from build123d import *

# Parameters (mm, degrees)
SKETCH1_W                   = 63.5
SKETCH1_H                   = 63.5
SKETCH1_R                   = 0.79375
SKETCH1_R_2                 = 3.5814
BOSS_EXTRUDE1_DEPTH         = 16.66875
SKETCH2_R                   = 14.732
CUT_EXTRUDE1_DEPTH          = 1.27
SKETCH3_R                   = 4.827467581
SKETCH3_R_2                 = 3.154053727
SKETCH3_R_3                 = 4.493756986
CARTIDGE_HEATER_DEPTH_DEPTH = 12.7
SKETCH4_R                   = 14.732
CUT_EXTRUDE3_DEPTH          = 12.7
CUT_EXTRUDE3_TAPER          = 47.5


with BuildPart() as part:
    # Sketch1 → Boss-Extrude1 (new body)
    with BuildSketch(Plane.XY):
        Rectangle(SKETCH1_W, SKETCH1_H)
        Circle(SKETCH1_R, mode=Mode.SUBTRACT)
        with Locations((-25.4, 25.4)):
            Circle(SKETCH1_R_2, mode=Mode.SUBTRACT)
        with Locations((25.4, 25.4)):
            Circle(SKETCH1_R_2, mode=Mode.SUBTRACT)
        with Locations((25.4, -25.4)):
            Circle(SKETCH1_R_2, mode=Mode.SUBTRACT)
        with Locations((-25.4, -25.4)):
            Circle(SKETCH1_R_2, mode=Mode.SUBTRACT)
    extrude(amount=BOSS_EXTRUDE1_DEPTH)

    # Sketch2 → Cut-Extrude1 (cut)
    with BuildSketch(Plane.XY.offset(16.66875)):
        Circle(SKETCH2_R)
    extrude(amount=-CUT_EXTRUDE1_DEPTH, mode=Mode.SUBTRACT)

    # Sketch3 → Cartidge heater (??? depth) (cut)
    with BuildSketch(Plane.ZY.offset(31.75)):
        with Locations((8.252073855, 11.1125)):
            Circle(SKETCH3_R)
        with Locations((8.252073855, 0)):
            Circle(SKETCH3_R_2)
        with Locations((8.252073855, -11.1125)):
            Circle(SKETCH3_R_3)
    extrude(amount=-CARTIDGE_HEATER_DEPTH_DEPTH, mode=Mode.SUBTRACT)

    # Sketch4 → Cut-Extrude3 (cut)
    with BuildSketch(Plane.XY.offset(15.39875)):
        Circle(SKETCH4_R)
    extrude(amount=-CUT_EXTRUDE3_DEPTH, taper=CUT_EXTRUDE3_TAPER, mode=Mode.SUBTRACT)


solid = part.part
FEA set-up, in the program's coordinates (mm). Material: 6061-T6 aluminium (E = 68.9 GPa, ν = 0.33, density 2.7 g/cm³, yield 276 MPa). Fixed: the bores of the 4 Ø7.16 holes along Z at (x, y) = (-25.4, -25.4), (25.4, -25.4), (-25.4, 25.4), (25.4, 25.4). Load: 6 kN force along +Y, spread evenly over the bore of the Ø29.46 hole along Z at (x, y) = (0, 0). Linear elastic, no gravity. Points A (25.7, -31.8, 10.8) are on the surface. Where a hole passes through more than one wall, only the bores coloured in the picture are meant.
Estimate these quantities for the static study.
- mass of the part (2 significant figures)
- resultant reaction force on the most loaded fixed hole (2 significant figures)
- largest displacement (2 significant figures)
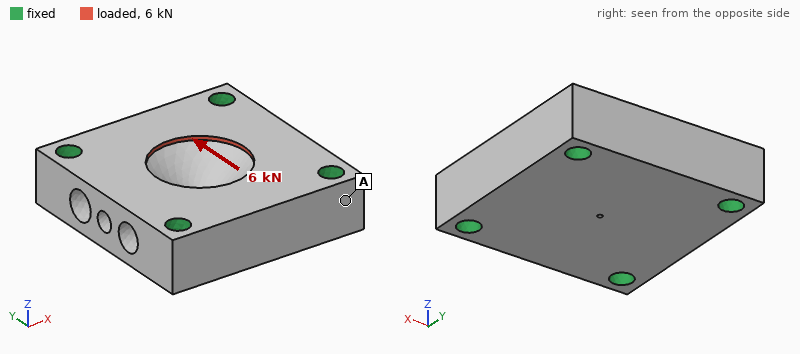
160 g
1.8 kN
5.9 µm
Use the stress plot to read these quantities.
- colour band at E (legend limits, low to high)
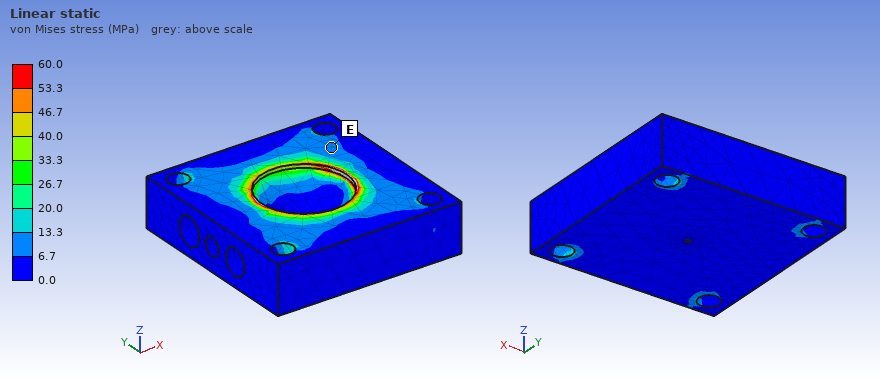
6.7 to 13.3 MPa
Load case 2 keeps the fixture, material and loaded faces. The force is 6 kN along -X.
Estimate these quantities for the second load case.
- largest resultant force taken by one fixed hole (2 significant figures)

1.7 kN
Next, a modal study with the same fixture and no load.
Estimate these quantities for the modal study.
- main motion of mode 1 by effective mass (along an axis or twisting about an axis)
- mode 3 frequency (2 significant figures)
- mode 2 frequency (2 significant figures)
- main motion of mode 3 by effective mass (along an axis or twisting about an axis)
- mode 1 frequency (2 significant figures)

along Z
24 kHz
22 kHz
twisting about X
17 kHz
